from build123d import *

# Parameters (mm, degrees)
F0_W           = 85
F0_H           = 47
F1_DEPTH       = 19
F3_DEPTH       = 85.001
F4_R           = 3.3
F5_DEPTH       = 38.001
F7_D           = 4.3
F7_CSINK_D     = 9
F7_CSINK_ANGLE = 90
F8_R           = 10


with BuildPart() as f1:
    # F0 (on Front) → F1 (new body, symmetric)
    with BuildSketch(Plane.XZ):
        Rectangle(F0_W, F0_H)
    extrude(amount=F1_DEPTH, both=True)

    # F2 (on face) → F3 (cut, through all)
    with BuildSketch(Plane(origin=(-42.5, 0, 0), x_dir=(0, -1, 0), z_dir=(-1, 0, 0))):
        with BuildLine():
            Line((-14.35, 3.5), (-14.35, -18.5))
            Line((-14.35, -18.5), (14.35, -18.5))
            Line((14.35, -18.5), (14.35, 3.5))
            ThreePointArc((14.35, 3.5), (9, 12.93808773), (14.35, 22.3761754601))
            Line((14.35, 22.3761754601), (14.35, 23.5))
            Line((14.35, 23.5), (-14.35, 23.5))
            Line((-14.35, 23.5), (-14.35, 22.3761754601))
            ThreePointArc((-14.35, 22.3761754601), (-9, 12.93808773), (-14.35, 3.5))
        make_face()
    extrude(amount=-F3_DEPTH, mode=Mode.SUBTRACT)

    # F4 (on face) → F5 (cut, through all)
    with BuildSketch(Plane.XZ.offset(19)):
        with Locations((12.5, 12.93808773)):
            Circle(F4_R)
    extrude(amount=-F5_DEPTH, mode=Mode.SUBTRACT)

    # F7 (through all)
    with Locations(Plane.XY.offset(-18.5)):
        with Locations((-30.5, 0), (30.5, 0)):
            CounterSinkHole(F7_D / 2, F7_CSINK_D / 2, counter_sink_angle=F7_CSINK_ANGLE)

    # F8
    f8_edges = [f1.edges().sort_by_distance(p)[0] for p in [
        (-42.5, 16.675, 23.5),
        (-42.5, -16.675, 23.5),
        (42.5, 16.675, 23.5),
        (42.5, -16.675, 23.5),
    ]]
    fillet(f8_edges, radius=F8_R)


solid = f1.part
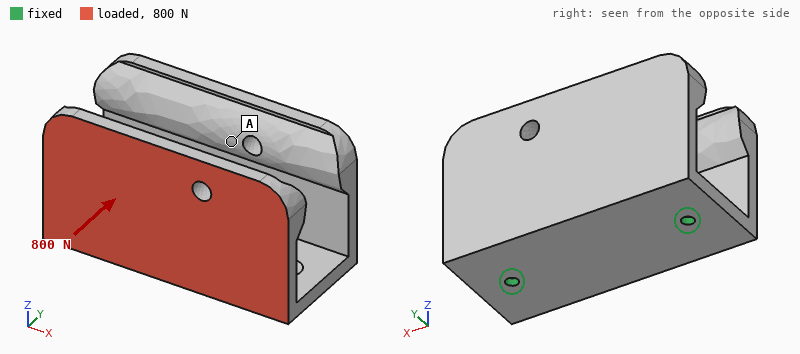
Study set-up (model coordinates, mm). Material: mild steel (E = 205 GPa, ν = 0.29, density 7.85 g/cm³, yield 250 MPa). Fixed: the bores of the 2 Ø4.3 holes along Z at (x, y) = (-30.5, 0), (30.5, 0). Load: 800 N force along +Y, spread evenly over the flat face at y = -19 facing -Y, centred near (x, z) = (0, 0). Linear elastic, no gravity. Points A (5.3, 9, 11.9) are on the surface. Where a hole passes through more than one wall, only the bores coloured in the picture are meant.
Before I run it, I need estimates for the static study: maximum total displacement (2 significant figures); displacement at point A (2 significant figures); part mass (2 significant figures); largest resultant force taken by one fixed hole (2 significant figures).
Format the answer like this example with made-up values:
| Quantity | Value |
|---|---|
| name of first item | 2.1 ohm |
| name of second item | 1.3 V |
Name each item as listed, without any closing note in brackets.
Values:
| Quantity | Value |
|---|---|
| maximum total displacement | 0.16 mm |
| displacement at point A | 0.040 mm |
| part mass | 470 g |
| largest resultant force taken by one fixed hole | 400 N |
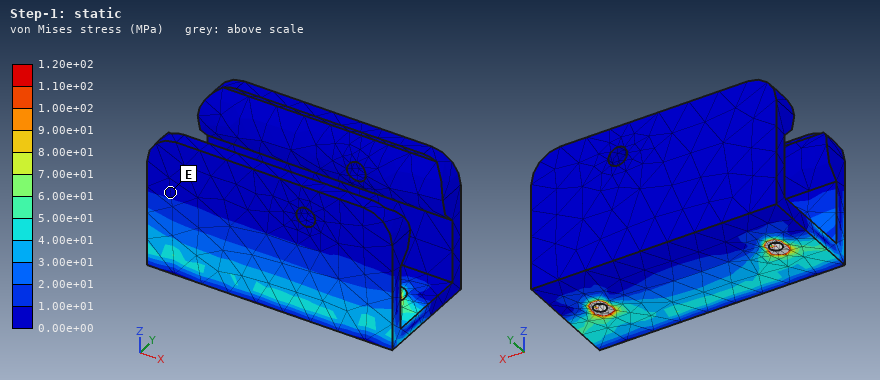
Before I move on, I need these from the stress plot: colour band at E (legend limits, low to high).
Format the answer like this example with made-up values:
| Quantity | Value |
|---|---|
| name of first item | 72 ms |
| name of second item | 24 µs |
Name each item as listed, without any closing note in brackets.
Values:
| Quantity | Value |
|---|---|
| colour band at E | 0.00e+00 to 1.00e+01 MPa |
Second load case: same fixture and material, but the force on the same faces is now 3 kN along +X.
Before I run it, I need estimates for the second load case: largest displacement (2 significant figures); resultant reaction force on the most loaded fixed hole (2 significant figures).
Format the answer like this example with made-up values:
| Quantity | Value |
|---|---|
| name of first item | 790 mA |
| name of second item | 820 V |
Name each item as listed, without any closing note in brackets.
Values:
| Quantity | Value |
|---|---|
| largest displacement | 51 µm |
| resultant reaction force on the most loaded fixed hole | 2.0 kN |
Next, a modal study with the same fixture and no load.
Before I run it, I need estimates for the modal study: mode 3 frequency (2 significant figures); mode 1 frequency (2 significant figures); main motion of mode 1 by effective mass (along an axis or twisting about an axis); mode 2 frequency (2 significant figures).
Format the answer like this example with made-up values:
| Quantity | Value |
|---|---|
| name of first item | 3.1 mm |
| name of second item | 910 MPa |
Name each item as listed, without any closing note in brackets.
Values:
| Quantity | Value |
|---|---|
| mode 3 frequency | 2000 Hz |
| mode 1 frequency | 740 Hz |
| main motion of mode 1 by effective mass | along Y |
| mode 2 frequency | 1100 Hz |
